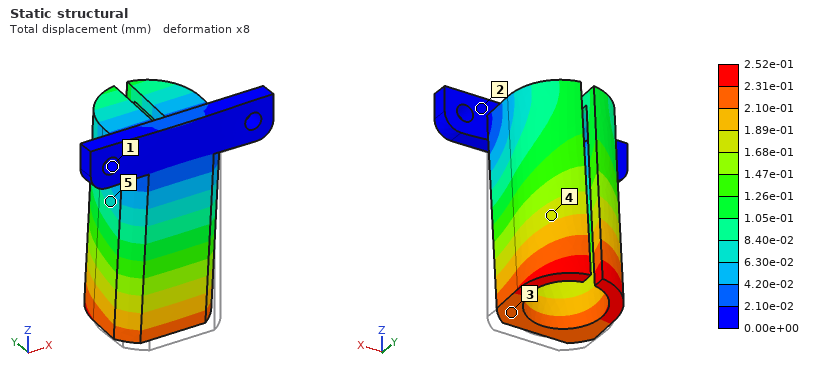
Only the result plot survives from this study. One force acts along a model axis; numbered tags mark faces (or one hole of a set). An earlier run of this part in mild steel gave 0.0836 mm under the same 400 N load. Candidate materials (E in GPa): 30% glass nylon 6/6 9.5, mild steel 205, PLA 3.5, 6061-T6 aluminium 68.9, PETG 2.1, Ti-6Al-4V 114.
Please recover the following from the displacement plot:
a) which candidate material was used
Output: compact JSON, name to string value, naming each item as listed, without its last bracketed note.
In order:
{"which candidate material was used": "6061-T6 aluminium"}
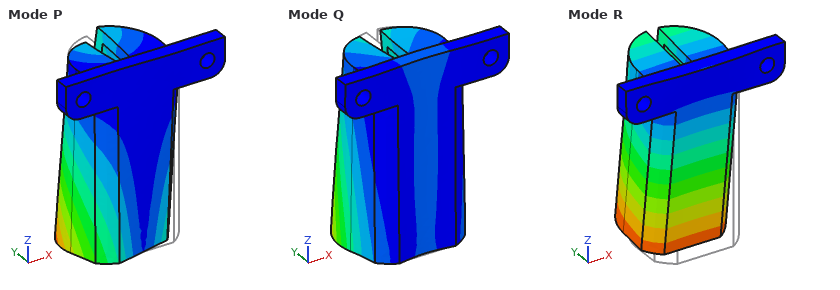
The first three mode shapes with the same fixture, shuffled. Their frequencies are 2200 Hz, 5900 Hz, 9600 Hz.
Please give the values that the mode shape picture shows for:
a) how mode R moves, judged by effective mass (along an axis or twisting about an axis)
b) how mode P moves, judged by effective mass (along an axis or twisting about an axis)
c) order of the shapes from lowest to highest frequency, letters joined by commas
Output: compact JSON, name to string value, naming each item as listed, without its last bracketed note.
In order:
{"how mode R moves, judged by effective mass": "along Y", "how mode P moves, judged by effective mass": "along X", "order of the shapes from lowest to highest frequency, letters joined by commas": "R, P, Q"}
